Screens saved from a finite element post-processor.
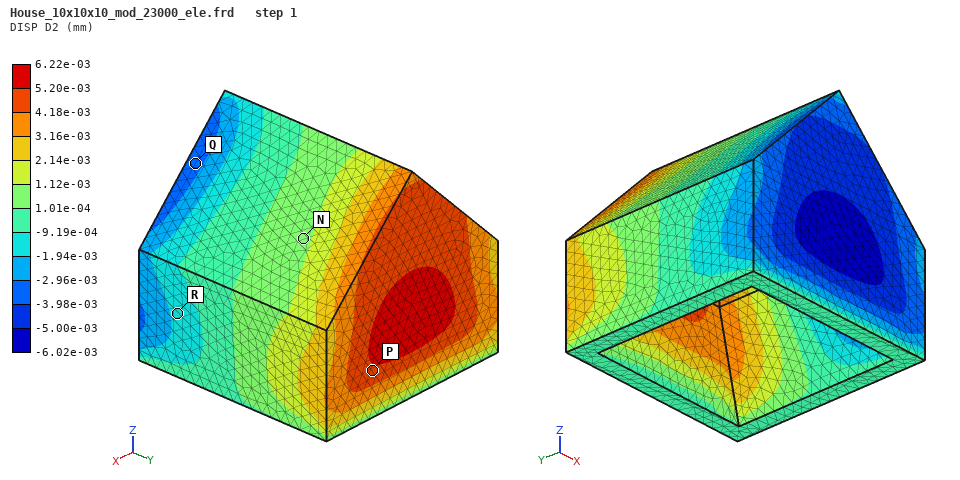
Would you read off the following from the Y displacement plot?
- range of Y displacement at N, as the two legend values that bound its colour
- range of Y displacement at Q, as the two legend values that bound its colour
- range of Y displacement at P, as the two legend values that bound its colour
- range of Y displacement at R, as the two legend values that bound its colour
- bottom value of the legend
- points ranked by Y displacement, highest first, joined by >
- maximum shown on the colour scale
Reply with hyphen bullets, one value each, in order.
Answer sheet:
- 1.01e-04 to 1.12e-03 mm
- -3.98e-03 to -2.96e-03 mm
- 4.18e-03 to 5.20e-03 mm
- -1.94e-03 to -9.19e-04 mm
- -6.02e-03 mm
- P > N > R > Q
- 6.22e-03 mm
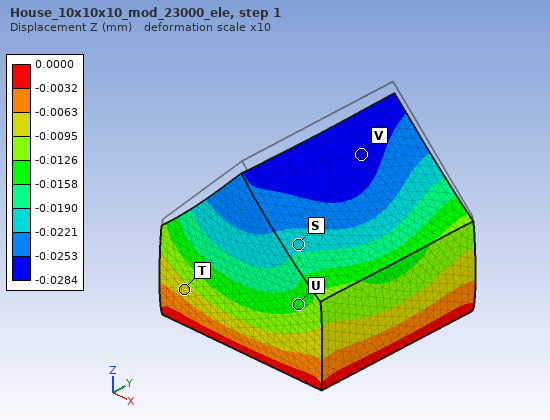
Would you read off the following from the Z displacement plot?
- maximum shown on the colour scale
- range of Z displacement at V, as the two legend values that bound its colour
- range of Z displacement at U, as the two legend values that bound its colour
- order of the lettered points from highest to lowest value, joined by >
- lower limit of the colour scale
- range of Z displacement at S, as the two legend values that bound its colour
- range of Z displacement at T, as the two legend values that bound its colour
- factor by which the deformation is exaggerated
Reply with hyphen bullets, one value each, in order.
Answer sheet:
- 0.0000 mm
- -0.0284 to -0.0253 mm
- -0.0158 to -0.0126 mm
- T > U > S > V
- -0.0284 mm
- -0.0221 to -0.0190 mm
- -0.0095 to -0.0063 mm
- 10
